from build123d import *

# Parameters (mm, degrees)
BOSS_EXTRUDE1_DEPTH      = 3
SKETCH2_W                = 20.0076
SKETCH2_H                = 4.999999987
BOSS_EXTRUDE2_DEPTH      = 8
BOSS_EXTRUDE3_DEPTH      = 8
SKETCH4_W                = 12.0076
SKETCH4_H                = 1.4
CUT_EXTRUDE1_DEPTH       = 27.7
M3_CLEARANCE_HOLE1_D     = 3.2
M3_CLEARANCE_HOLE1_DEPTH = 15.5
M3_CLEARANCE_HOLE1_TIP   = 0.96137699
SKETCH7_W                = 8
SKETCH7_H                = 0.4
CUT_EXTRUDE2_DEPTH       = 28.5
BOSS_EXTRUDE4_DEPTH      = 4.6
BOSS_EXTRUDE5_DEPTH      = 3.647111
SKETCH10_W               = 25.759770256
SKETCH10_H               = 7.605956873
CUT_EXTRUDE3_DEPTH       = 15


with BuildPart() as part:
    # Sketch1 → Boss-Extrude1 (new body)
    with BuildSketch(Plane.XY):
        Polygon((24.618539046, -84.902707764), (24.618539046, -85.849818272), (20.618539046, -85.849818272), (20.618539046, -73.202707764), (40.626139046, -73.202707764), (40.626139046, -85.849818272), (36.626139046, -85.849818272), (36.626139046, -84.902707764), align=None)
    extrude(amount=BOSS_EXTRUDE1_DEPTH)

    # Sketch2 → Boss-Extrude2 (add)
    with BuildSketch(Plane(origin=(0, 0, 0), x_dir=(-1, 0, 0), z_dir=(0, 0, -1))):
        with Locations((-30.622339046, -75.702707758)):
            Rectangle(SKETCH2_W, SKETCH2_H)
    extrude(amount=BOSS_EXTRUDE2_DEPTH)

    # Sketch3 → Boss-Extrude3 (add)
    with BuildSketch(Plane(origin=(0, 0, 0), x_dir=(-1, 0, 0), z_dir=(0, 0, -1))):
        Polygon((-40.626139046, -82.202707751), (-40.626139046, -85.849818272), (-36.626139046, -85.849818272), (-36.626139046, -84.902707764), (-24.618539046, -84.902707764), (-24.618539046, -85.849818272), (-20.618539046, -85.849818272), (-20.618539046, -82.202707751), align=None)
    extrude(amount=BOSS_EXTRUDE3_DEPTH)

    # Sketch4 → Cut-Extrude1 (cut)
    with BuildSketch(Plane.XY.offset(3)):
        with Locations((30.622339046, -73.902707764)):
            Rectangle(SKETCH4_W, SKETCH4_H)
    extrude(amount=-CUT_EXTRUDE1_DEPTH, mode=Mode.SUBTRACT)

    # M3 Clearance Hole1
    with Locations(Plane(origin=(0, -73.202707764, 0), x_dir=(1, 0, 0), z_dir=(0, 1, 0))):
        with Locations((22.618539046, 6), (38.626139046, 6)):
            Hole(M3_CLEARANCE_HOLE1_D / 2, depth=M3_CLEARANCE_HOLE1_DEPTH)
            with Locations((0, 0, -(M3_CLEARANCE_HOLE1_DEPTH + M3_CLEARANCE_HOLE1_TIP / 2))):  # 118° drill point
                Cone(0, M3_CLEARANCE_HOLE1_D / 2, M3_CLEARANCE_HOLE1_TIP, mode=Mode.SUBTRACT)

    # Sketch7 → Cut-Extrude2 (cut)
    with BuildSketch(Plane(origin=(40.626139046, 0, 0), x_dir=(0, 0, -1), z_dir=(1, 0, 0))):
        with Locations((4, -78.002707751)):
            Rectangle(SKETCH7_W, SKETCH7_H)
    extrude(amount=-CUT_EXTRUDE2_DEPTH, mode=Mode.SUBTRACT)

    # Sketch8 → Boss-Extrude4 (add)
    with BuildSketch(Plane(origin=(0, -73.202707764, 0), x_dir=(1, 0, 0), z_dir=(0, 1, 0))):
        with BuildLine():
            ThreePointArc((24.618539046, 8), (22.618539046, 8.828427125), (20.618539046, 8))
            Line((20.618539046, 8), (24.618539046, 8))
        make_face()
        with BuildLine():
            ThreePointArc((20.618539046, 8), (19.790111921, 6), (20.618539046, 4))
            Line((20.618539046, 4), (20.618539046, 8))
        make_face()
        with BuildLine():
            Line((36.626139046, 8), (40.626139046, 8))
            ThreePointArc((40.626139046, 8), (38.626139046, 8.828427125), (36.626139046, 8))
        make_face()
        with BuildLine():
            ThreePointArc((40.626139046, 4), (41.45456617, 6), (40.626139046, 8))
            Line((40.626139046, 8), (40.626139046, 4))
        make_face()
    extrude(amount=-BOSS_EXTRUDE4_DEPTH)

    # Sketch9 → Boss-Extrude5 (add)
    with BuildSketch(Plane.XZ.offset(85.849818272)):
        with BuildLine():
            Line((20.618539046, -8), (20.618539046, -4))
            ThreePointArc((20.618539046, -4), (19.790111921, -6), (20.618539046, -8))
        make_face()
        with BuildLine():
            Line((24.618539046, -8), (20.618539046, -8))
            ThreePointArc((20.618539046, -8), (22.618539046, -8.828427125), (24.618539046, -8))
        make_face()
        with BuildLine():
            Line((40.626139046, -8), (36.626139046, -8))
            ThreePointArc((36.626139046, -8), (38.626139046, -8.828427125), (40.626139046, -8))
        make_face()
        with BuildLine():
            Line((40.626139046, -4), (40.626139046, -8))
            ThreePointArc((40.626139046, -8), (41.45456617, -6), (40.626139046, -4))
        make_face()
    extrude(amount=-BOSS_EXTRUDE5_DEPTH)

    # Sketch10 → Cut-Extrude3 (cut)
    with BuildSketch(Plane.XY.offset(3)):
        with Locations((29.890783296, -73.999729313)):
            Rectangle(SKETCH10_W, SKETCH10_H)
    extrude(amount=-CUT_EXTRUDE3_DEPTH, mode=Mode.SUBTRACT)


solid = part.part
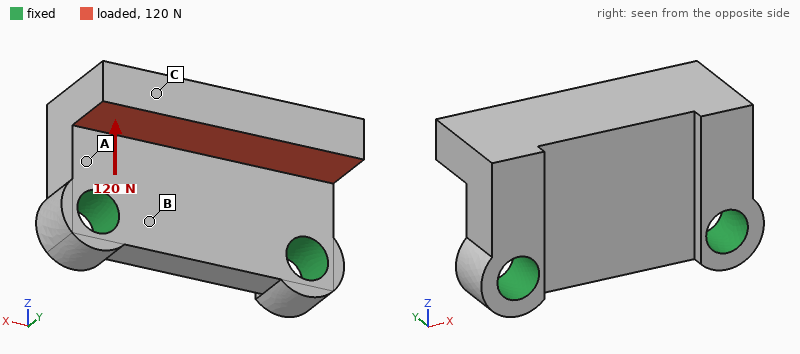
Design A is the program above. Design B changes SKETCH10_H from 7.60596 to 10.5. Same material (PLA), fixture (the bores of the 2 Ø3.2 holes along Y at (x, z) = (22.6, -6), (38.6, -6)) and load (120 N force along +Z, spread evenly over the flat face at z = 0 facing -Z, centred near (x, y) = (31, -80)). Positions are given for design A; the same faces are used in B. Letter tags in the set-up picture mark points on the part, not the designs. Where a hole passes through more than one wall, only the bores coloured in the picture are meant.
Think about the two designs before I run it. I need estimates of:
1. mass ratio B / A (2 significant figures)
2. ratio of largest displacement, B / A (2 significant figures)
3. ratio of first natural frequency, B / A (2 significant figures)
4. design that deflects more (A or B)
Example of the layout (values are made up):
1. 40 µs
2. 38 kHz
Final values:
1. 0.91
2. 0.70
3. 1.2
4. A
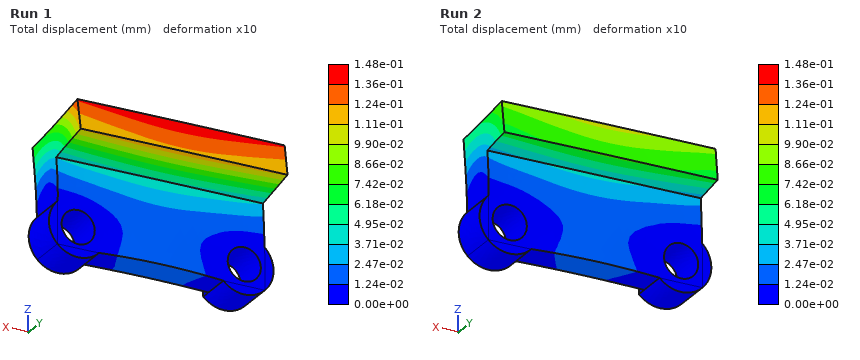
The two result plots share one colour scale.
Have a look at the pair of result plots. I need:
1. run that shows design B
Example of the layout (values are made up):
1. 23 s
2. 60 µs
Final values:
1. Run 2
